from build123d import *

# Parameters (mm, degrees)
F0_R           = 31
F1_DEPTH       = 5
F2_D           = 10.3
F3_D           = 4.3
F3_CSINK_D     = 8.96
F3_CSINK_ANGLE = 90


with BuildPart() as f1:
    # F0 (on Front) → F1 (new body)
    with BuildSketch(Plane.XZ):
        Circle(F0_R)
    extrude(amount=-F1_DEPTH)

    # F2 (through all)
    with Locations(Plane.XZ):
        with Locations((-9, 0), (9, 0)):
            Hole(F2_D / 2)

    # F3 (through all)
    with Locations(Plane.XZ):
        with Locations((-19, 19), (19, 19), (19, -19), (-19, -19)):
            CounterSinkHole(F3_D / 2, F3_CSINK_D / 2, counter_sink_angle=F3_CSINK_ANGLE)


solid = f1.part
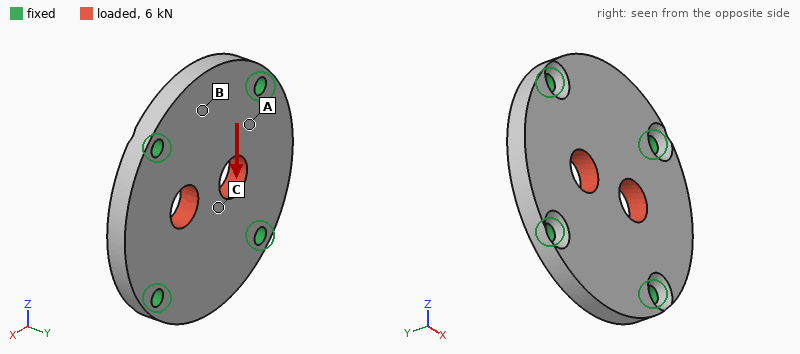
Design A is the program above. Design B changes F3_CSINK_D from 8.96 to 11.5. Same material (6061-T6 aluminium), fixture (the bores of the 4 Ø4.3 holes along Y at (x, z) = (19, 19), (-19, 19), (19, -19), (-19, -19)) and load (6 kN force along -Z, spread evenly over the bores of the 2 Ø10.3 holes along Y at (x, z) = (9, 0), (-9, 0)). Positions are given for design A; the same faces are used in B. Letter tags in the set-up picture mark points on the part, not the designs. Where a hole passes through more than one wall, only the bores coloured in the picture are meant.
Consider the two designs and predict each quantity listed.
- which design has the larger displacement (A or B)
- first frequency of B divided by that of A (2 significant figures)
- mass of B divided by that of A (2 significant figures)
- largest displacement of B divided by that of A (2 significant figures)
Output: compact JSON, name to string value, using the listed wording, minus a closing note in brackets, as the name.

{"which design has the larger displacement": "B", "first frequency of B divided by that of A": "0.92", "mass of B divided by that of A": "0.98", "largest displacement of B divided by that of A": "1.2"}
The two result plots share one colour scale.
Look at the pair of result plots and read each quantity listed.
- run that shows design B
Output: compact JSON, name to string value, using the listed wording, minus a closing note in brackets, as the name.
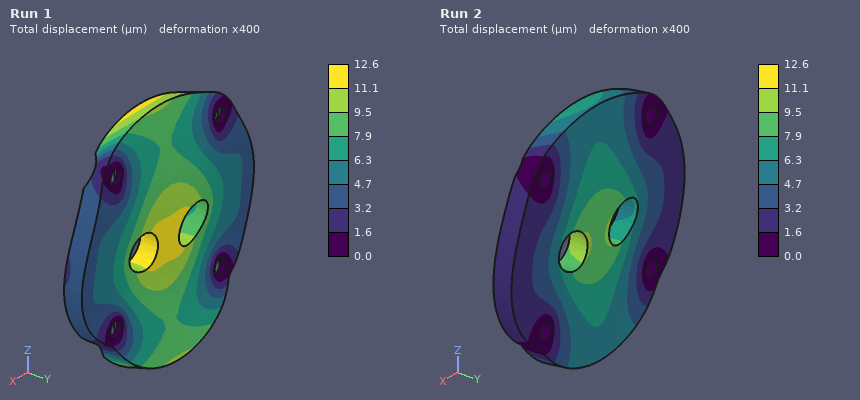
{"run that shows design B": "Run 1"}
